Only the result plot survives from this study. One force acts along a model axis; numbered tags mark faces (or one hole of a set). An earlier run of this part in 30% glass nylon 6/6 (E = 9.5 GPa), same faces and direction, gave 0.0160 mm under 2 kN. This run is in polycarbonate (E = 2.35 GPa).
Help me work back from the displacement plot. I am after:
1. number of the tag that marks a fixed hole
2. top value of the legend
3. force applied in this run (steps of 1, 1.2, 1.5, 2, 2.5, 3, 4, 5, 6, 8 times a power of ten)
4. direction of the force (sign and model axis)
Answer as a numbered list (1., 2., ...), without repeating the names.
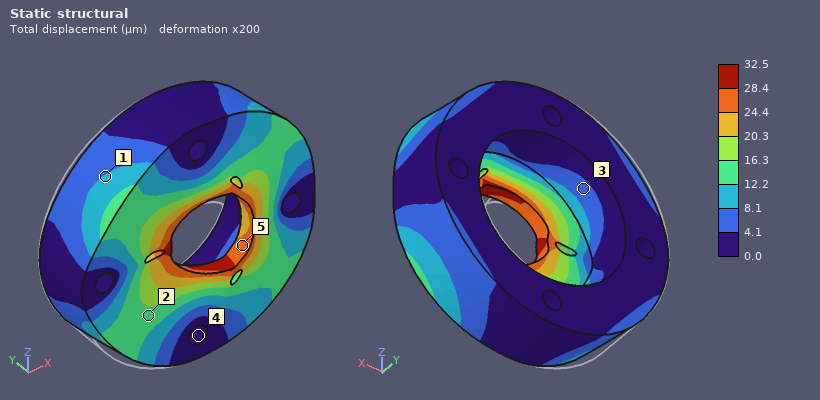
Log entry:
1. 4
2. 32.5 µm
3. 1 kN
4. +X
